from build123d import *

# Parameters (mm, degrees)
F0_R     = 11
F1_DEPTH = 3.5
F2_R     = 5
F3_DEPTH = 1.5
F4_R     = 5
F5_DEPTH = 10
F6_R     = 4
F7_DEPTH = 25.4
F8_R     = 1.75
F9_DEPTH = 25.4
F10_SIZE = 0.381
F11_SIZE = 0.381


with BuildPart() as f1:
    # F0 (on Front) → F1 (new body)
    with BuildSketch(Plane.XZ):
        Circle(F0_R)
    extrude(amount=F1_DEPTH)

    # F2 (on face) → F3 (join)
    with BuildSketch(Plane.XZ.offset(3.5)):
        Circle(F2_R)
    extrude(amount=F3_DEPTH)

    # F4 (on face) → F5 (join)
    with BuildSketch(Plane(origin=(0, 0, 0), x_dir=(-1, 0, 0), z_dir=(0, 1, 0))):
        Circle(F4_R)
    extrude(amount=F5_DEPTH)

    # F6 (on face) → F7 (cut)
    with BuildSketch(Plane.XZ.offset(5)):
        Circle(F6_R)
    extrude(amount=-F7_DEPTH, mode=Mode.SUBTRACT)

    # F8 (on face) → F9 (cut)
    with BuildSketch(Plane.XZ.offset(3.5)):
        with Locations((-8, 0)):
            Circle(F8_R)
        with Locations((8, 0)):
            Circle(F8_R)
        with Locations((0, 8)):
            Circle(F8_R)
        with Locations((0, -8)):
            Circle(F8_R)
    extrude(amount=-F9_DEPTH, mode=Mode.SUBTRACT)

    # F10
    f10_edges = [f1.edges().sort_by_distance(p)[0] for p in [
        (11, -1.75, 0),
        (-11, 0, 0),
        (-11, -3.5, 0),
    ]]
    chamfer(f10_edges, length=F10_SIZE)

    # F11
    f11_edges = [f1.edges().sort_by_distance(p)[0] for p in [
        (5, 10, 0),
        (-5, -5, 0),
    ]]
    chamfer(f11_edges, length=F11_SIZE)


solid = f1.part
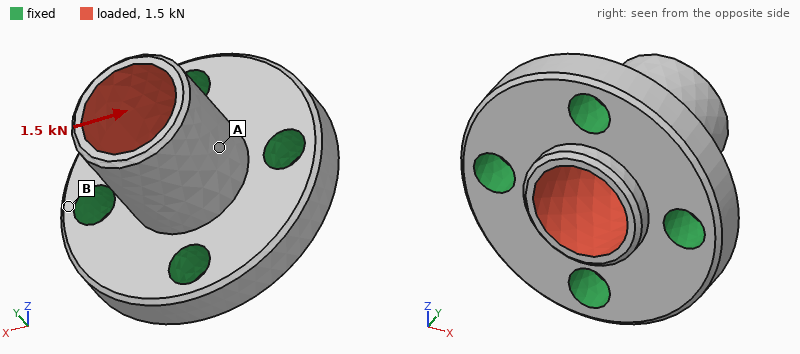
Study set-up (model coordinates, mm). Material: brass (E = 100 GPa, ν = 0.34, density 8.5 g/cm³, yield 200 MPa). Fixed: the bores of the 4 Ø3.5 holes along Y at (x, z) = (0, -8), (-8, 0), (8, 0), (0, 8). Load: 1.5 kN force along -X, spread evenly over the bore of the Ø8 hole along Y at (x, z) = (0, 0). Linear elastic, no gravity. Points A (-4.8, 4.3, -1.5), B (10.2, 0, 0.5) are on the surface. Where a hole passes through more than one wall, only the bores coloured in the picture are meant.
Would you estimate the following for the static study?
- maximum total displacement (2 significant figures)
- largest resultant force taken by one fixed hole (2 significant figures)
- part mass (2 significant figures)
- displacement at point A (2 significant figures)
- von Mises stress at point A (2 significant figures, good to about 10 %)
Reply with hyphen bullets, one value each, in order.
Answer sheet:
- 20 µm
- 630 N
- 11 g
- 12 µm
- 33 MPa
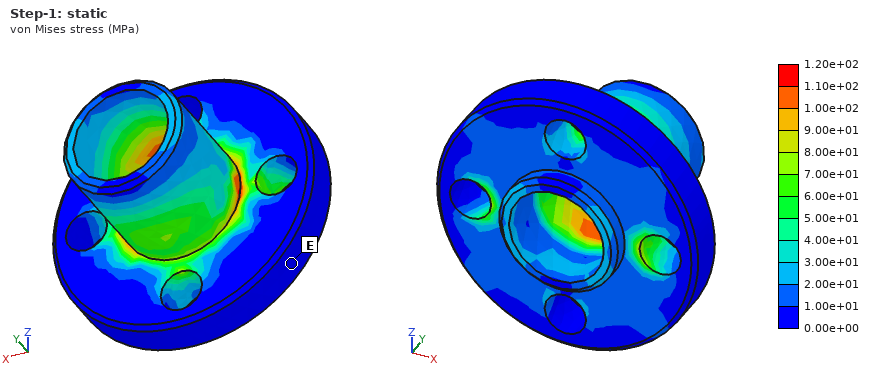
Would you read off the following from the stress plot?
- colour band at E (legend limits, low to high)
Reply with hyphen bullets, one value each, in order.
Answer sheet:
- 0.00e+00 to 1.00e+01 MPa
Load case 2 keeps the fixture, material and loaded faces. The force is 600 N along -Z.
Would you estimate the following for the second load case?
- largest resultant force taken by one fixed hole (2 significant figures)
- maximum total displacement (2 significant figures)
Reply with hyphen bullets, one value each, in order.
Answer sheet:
- 250 N
- 7.9 µm
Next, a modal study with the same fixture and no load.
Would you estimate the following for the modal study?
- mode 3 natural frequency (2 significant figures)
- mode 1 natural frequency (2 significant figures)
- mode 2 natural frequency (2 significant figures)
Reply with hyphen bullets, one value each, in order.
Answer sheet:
- 27 kHz
- 27 kHz
- 27 kHz
